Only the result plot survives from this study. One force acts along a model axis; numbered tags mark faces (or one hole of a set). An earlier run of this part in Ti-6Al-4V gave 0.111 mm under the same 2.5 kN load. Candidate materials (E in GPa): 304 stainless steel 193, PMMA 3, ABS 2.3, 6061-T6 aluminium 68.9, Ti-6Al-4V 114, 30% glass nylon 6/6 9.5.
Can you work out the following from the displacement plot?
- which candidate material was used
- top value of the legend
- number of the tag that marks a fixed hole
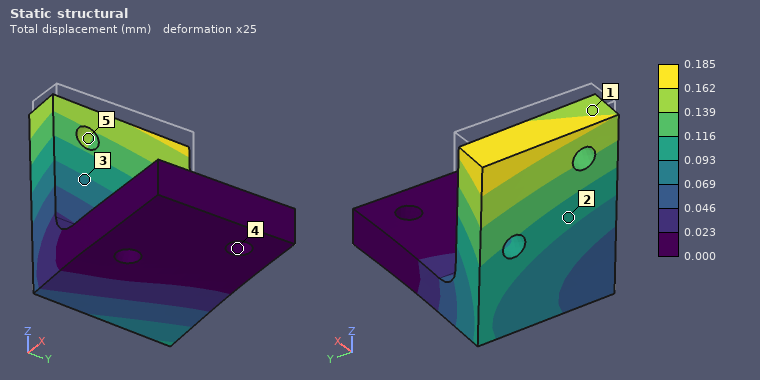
6061-T6 aluminium
0.185 mm
4
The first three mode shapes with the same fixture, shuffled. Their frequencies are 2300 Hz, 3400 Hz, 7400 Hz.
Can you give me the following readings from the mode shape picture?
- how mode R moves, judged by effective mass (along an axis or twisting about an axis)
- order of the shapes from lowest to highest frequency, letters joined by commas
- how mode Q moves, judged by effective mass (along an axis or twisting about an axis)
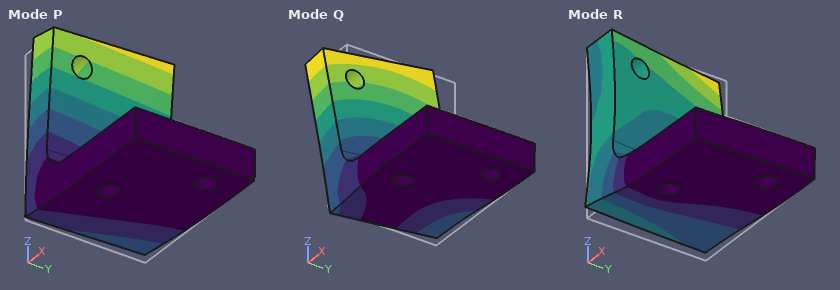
along Z
P, Q, R
along Y
